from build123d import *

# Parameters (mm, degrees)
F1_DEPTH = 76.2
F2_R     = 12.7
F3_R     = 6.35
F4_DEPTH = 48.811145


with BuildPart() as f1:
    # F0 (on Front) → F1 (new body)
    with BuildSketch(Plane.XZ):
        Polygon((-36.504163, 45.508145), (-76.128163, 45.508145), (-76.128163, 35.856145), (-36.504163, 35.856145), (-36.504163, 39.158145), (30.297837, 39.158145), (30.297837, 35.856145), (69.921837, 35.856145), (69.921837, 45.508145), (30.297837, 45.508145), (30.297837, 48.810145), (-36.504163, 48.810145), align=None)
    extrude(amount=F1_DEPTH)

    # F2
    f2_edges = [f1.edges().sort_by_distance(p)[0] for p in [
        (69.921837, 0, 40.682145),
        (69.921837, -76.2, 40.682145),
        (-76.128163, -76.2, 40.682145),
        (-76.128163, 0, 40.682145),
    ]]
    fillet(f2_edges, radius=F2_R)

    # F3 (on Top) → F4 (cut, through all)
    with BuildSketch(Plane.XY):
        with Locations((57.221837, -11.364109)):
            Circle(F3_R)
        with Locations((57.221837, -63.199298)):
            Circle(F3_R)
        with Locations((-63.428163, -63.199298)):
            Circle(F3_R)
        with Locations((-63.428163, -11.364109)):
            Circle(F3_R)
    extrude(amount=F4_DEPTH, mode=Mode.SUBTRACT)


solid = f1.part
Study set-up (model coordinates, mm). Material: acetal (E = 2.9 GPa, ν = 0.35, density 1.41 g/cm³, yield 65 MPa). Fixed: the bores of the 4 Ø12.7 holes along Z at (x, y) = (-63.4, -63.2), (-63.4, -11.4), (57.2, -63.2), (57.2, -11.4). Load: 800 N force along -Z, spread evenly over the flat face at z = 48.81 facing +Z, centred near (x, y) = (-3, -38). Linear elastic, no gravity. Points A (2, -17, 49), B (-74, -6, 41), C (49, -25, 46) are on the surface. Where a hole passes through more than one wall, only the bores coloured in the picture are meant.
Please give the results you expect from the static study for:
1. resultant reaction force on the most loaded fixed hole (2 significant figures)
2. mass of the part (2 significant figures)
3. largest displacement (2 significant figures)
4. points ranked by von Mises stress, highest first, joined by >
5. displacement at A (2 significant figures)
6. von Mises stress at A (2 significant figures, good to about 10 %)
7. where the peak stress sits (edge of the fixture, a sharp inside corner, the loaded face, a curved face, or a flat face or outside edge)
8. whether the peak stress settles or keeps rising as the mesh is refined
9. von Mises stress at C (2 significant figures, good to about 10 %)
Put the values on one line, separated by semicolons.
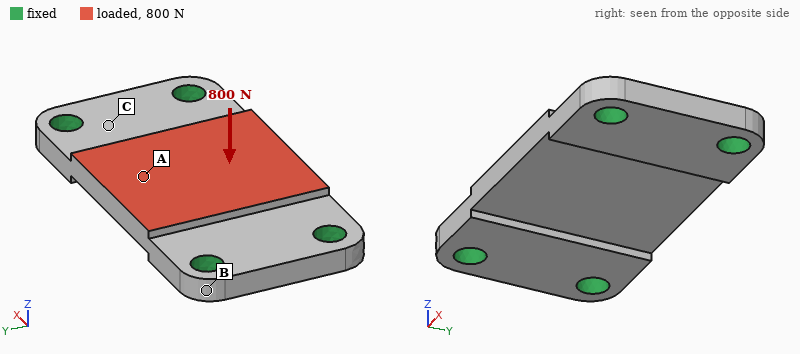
400 N; 140 g; 0.27 mm; A > C > B; 0.25 mm; 4.8 MPa; edge of the fixture; keeps rising; 2.7 MPa
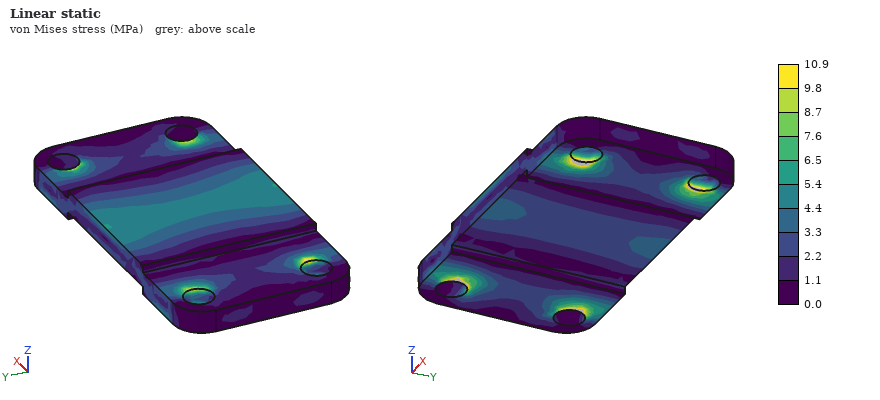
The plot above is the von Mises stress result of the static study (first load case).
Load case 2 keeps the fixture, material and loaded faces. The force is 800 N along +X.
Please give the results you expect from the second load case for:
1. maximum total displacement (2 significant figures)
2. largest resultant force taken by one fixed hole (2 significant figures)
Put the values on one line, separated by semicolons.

11 µm; 210 N
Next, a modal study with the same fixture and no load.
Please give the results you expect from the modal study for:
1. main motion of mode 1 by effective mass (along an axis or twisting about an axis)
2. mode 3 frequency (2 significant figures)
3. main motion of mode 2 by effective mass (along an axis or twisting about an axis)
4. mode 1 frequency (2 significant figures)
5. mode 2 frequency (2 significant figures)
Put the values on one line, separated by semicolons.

along Z; 2500 Hz; twisting about X; 1100 Hz; 1500 Hz
